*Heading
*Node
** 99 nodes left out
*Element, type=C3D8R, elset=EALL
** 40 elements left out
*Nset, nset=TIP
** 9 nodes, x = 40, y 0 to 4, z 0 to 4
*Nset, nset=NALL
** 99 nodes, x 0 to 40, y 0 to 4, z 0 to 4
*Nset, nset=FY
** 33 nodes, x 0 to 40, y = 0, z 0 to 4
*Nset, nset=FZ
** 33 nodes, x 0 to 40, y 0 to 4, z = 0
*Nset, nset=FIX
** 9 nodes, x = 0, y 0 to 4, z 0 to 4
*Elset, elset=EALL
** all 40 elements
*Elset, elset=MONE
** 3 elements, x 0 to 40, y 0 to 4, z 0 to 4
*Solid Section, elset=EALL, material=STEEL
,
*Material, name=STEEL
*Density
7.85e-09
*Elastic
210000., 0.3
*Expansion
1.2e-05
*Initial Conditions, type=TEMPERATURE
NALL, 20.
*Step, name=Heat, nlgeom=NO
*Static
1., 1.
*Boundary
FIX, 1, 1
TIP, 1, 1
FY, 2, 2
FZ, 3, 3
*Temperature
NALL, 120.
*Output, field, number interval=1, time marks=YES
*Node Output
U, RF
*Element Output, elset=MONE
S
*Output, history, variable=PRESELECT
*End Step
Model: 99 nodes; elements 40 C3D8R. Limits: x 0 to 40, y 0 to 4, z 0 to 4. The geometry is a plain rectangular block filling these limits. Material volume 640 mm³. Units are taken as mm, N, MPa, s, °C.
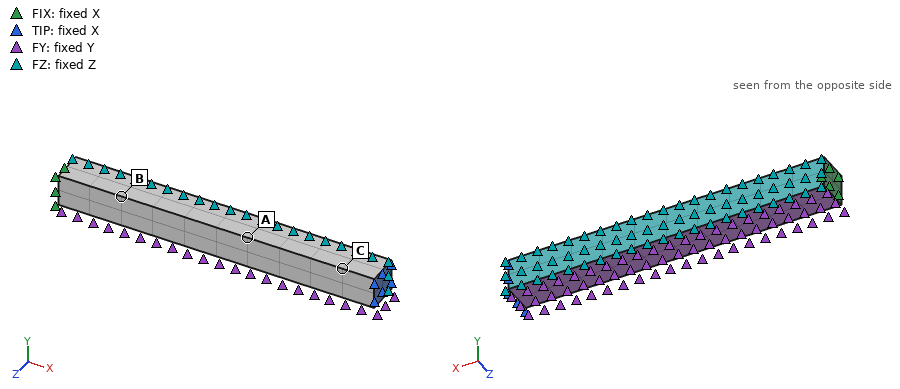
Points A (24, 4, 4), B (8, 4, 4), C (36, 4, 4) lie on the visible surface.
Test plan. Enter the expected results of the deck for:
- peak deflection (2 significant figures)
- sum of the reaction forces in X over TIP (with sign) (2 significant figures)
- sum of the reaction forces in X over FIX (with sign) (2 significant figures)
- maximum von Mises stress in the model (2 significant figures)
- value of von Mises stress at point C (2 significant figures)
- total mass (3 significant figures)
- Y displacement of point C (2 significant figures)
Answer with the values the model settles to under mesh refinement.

0.0088 mm
-4000 N
4000 N
250 MPa
250 MPa
0.00502 kg
0.0062 mm
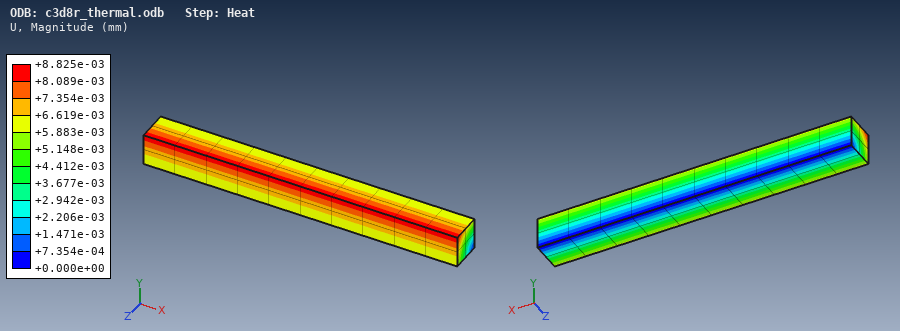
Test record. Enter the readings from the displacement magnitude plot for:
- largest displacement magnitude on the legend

+8.825e-03 mm
